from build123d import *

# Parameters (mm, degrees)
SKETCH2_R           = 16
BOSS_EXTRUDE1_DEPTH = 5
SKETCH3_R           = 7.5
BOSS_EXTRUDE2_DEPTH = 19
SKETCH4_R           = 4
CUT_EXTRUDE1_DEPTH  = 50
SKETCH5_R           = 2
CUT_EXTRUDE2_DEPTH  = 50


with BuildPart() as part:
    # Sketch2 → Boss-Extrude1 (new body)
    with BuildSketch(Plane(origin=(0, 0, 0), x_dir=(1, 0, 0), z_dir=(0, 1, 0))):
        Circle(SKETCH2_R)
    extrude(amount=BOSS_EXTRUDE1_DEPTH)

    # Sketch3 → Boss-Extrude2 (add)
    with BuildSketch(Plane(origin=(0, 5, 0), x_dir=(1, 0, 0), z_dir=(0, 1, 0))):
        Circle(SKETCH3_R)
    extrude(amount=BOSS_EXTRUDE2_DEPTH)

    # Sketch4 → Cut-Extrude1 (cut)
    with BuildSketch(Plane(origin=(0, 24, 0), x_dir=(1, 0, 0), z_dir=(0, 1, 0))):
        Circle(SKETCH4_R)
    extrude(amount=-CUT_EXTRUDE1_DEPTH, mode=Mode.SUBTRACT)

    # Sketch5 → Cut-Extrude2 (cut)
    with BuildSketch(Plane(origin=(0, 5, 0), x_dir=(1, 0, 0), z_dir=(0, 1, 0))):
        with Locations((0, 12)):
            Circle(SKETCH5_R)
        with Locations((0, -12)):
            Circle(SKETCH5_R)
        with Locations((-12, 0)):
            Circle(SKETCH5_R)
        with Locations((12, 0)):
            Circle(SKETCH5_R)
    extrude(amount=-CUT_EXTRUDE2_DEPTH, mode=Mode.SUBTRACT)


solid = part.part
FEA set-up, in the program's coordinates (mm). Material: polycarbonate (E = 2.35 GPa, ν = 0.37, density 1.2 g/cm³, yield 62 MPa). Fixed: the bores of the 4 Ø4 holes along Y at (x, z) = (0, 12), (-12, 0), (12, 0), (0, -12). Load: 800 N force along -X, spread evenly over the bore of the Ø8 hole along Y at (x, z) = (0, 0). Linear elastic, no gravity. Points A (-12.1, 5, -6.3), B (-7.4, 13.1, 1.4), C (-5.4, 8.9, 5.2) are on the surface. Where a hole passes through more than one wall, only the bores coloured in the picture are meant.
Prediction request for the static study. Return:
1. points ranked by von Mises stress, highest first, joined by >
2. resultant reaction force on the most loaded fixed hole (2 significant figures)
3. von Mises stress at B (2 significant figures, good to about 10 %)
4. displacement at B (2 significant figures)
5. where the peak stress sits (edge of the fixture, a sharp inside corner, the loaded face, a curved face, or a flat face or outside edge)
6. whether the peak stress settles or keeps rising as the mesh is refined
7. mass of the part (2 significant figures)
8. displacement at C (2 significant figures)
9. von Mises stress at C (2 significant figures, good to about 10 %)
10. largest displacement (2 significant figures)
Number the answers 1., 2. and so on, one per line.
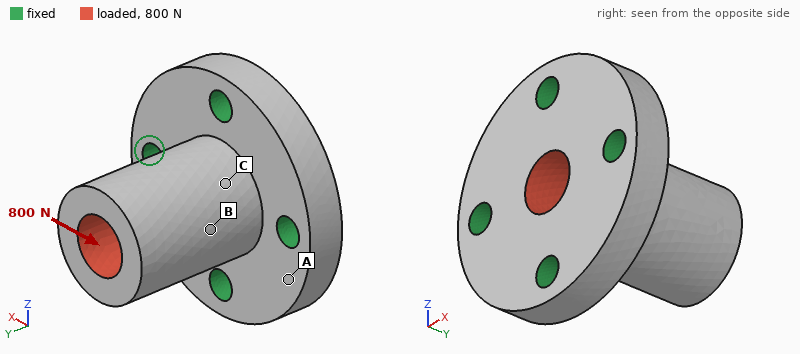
1. C > B > A
2. 450 N
3. 5.6 MPa
4. 0.19 mm
5. edge of the fixture
6. keeps rising
7. 7.1 g
8. 0.11 mm
9. 11 MPa
10. 0.36 mm
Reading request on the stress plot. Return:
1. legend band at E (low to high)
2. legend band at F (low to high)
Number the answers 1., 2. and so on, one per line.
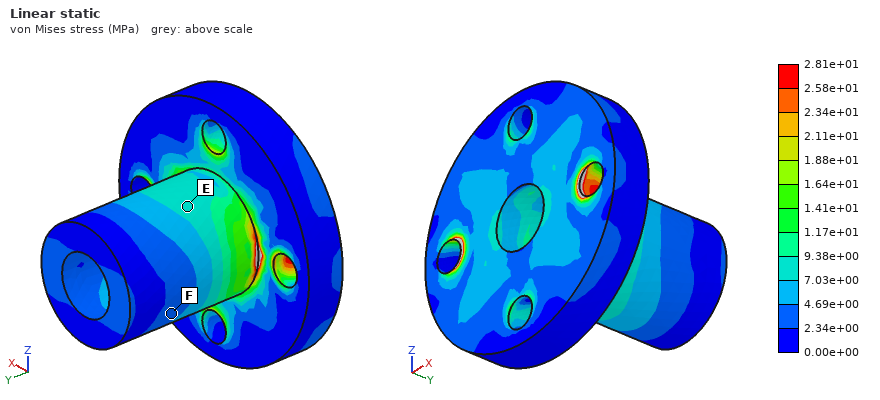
1. 7.03e+00 to 9.38e+00 MPa
2. 2.34e+00 to 4.69e+00 MPa
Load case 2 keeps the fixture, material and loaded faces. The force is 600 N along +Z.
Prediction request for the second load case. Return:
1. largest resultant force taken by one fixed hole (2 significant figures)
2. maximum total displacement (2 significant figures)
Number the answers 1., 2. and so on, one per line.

1. 330 N
2. 0.27 mm
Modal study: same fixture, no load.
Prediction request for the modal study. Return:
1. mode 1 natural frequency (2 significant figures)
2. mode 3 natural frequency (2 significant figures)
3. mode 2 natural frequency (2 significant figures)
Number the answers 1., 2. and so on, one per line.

1. 4700 Hz
2. 10 kHz
3. 4700 Hz
